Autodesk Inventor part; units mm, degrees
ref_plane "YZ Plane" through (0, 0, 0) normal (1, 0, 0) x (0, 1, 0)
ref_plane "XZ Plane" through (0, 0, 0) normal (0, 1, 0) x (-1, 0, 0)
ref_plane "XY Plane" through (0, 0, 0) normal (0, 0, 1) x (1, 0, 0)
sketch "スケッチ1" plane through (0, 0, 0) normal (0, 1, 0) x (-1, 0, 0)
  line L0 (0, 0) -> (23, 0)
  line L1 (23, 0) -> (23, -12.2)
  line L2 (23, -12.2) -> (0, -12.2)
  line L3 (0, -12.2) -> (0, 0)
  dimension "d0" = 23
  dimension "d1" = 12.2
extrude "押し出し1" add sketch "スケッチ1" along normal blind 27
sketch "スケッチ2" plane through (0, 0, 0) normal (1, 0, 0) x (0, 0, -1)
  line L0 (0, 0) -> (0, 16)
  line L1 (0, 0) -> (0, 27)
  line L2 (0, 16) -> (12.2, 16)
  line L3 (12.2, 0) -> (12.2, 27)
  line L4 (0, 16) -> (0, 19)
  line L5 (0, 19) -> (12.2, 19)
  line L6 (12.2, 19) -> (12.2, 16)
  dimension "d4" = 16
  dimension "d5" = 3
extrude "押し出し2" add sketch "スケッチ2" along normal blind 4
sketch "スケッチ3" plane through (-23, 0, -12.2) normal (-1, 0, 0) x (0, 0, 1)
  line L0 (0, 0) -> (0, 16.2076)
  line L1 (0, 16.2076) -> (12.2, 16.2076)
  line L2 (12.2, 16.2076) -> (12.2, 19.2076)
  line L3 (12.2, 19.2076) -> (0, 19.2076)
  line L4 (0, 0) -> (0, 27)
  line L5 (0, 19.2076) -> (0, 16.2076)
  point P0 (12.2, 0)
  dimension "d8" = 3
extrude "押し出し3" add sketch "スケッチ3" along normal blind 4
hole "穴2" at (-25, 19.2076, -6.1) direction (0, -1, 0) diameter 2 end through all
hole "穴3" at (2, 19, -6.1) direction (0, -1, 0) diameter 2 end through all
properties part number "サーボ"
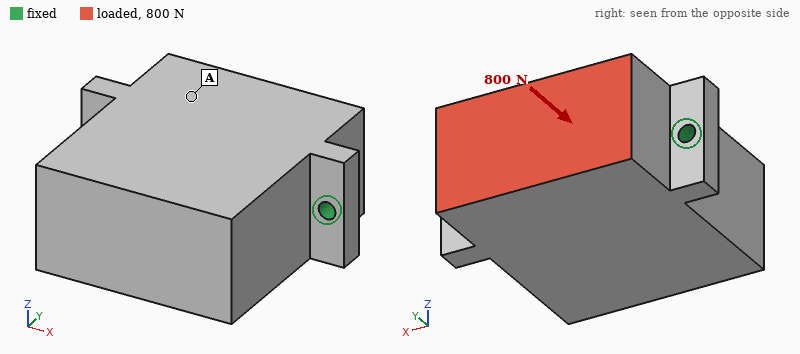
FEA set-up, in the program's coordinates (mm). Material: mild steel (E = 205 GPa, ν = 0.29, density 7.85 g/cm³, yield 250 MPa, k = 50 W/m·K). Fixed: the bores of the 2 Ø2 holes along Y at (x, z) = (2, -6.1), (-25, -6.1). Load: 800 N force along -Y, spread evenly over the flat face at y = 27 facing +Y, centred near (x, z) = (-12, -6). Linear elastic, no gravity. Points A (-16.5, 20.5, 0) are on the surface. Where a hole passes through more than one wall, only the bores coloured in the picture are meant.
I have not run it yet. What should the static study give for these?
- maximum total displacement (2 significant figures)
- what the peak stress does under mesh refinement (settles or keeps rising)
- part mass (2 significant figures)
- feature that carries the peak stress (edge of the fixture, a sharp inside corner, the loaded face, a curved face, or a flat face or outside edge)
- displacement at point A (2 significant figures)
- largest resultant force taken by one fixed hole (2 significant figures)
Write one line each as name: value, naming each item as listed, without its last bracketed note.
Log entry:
maximum total displacement: 1.2 µm
what the peak stress does under mesh refinement: keeps rising
part mass: 62 g
feature that carries the peak stress: edge of the fixture
displacement at point A: 1.1 µm
largest resultant force taken by one fixed hole: 400 N
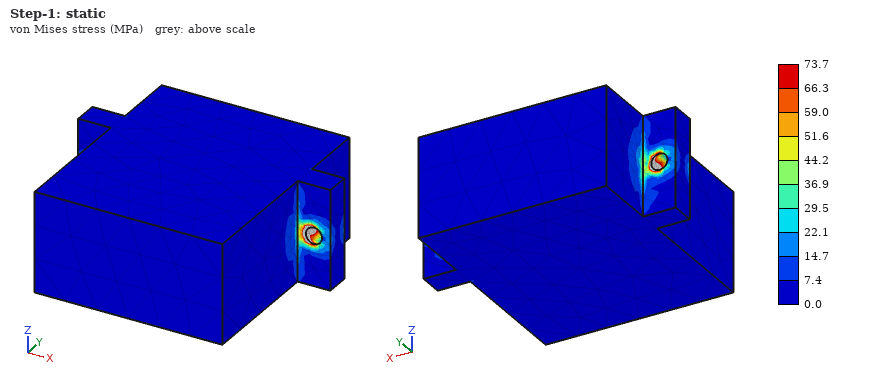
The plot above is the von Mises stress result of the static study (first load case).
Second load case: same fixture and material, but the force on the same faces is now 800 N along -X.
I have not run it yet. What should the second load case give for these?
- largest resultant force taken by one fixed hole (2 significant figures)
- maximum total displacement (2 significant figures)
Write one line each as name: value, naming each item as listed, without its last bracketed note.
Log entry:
largest resultant force taken by one fixed hole: 500 N
maximum total displacement: 1.6 µm
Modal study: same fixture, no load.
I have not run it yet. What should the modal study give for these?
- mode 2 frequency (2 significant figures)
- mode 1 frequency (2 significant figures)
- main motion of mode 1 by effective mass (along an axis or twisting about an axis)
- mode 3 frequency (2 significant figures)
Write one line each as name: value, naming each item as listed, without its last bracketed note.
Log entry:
mode 2 frequency: 18 kHz
mode 1 frequency: 4600 Hz
main motion of mode 1 by effective mass: along Z
mode 3 frequency: 18 kHz
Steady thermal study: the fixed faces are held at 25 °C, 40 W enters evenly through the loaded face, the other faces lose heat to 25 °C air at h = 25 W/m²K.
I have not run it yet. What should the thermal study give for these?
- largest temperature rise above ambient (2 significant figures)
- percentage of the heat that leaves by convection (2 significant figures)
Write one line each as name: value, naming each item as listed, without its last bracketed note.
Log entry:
largest temperature rise above ambient: 77 K
percentage of the heat that leaves by convection: 7.2 %
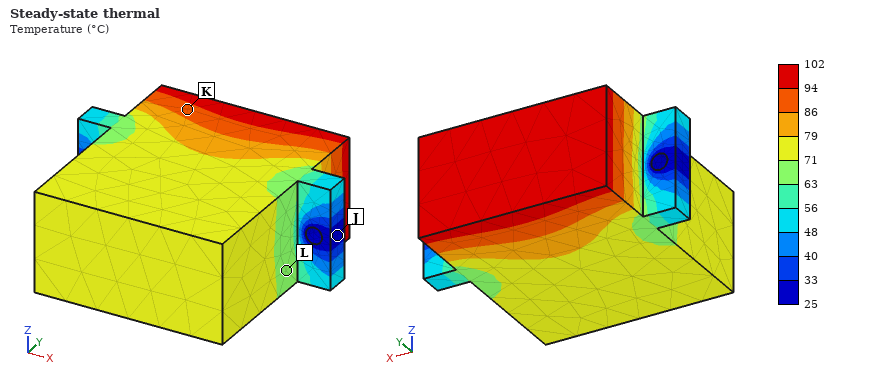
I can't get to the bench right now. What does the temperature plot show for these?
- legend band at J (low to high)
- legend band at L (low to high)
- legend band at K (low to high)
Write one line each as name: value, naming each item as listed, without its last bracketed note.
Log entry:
legend band at J: 25 to 33 °C
legend band at L: 63 to 71 °C
legend band at K: 86 to 94 °C
